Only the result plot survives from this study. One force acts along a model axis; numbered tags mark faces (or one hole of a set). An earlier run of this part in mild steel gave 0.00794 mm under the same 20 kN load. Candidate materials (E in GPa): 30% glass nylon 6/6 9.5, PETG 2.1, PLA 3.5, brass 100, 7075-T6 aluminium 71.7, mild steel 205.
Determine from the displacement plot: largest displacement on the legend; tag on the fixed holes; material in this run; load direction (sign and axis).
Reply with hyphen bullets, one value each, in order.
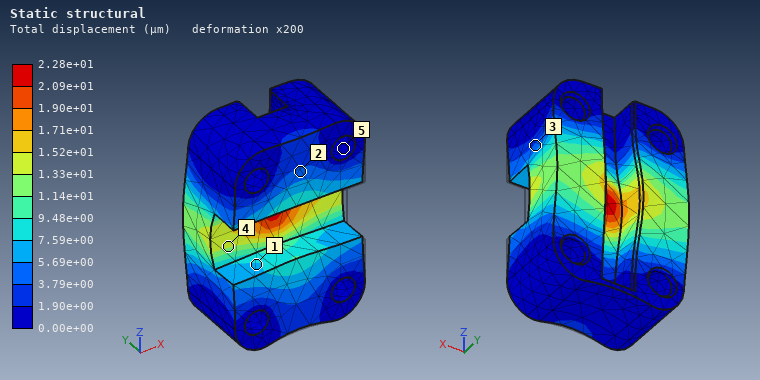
- 2.28e+01 µm
- 5
- 7075-T6 aluminium
- +Y
